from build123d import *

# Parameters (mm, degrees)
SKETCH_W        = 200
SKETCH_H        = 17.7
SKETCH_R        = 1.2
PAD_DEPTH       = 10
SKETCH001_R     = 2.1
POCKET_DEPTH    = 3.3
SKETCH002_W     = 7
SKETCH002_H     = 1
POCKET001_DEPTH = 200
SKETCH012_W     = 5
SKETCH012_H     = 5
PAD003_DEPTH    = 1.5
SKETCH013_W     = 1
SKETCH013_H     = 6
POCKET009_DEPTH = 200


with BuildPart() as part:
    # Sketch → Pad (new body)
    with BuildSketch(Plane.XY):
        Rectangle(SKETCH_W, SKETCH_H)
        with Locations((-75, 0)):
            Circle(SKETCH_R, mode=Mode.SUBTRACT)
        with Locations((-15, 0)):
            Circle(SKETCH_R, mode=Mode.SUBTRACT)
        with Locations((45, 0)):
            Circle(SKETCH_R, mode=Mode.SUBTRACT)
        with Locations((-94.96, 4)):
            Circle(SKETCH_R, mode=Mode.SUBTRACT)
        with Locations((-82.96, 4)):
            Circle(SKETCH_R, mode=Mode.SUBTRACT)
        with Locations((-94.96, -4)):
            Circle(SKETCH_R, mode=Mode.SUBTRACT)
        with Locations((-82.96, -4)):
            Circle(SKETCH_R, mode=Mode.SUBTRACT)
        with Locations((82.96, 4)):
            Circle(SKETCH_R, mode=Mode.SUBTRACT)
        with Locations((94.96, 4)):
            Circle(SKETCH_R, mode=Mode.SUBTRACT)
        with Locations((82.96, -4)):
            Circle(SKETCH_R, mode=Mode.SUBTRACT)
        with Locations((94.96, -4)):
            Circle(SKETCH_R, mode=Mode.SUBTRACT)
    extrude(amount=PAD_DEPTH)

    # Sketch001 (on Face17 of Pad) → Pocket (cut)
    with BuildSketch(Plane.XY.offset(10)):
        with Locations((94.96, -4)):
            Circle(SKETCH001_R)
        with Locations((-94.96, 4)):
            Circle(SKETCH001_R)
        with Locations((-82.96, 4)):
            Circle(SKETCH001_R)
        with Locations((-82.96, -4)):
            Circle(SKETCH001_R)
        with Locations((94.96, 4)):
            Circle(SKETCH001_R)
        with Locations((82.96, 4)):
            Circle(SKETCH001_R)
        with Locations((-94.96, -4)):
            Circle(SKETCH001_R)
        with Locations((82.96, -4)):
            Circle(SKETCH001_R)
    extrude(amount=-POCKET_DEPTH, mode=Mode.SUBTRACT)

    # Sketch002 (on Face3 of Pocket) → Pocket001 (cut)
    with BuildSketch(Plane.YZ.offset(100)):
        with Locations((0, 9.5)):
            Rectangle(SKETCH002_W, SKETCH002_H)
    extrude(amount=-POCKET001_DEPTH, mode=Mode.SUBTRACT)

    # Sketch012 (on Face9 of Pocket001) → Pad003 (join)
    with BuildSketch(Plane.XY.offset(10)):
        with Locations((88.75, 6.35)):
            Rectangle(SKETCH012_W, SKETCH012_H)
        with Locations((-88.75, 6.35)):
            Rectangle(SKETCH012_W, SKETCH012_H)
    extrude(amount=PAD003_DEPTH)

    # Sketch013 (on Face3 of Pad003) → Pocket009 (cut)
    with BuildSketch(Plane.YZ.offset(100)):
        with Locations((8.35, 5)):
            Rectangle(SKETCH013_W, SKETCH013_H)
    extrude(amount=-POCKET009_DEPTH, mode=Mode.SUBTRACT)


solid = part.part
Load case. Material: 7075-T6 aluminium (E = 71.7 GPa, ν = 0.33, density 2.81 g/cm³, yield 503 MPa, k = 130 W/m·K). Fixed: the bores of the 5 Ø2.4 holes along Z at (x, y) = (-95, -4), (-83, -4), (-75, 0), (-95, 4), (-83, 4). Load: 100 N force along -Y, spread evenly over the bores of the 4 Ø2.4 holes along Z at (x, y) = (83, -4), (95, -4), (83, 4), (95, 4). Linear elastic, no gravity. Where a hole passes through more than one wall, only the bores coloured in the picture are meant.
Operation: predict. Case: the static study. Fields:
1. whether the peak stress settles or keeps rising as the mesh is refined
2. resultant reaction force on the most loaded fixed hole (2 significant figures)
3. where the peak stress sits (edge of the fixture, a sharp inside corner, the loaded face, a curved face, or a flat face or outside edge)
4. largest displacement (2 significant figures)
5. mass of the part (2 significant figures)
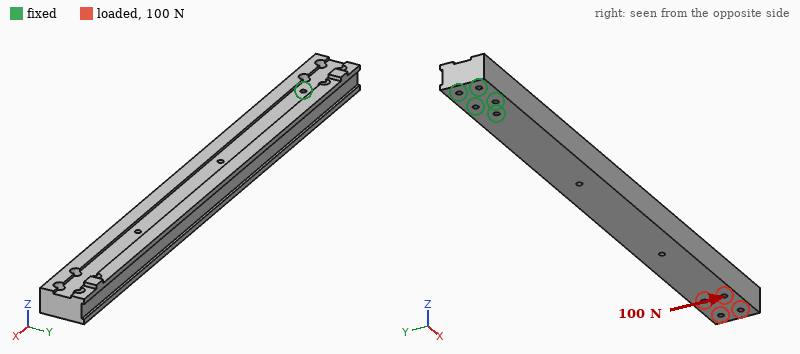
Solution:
keeps rising
810 N
edge of the fixture
0.62 mm
90 g
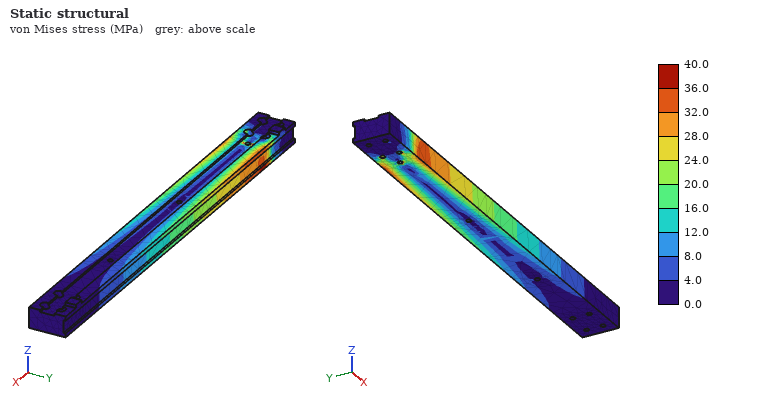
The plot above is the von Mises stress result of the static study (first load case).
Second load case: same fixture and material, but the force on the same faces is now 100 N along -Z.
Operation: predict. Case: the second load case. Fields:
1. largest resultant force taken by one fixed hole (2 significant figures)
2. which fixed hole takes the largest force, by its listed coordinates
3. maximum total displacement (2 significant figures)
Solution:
800 N
(-75, 0)
1.8 mm
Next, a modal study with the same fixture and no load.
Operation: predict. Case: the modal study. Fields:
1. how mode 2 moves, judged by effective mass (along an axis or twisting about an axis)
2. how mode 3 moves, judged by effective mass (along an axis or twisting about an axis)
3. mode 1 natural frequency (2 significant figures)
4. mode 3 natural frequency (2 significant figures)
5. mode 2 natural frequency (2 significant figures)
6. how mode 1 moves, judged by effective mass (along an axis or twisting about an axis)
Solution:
along Y
along Z
260 Hz
1600 Hz
430 Hz
along Z
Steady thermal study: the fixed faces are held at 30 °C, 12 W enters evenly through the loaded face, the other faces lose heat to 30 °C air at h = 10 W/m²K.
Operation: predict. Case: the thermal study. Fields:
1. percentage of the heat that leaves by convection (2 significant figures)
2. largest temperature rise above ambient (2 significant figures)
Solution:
33 %
72 K
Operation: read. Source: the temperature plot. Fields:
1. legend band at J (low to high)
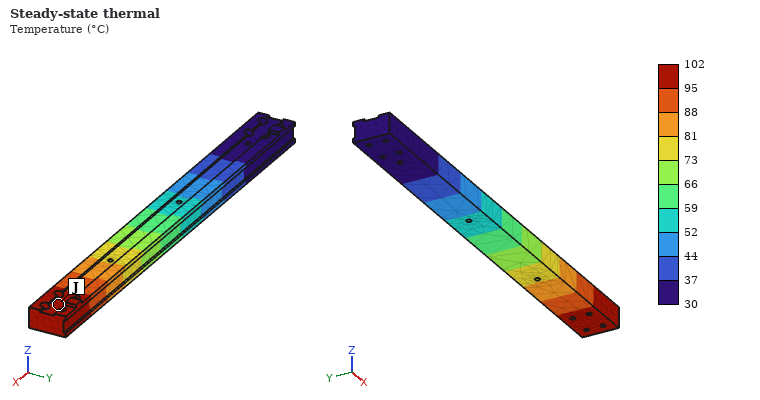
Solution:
95 to 102 °C
